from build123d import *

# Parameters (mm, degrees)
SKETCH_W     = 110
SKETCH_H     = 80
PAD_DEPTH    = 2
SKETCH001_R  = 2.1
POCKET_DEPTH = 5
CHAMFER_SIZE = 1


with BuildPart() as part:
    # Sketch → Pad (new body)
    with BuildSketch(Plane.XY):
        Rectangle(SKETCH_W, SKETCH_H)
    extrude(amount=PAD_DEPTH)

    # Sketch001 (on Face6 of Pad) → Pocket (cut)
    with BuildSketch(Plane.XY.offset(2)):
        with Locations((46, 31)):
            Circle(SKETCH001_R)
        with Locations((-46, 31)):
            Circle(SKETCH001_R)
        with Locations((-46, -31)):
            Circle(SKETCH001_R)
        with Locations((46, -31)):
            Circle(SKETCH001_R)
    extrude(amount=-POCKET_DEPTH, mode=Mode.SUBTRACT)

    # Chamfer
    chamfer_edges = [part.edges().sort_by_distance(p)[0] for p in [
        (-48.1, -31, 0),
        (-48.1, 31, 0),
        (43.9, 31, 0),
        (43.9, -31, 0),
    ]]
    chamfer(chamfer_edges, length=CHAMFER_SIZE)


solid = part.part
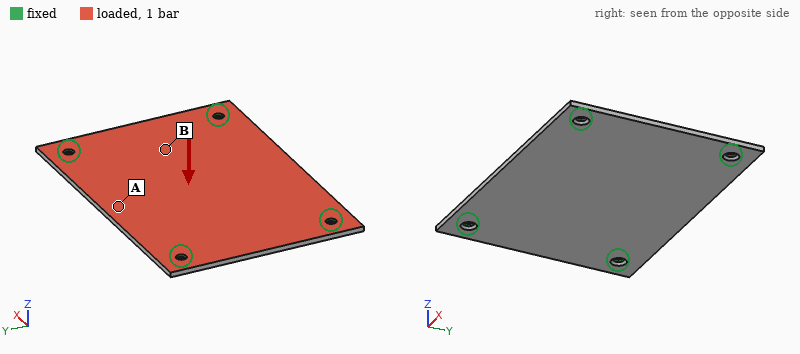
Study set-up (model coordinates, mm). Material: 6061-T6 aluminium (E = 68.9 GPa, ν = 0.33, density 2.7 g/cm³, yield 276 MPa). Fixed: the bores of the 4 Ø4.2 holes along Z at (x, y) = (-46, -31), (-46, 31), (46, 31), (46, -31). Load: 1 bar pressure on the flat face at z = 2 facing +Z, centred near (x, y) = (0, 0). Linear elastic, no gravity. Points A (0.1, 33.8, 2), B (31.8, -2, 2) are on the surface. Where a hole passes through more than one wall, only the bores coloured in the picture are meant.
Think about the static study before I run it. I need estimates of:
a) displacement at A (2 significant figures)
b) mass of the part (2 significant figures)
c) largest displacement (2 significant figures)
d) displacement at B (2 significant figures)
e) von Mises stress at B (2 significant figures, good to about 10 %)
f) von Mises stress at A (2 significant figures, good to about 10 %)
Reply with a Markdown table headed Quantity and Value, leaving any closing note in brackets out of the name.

| Quantity | Value |
|---|---|
| displacement at A | 0.57 mm |
| mass of the part | 47 g |
| largest displacement | 0.65 mm |
| displacement at B | 0.34 mm |
| von Mises stress at B | 31 MPa |
| von Mises stress at A | 64 MPa |
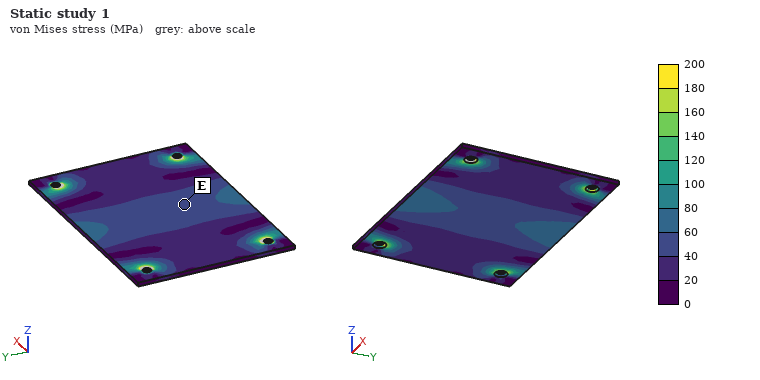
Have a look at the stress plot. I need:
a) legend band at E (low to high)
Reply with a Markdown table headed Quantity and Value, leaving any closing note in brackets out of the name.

| Quantity | Value |
|---|---|
| legend band at E | 40 to 60 MPa |
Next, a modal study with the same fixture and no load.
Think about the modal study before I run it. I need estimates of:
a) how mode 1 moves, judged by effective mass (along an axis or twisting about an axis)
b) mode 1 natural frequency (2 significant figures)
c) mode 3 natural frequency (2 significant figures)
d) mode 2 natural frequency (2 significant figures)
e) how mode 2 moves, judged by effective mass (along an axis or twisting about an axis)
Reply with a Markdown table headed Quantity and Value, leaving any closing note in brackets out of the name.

| Quantity | Value |
|---|---|
| how mode 1 moves, judged by effective mass | along Z |
| mode 1 natural frequency | 990 Hz |
| mode 3 natural frequency | 2300 Hz |
| mode 2 natural frequency | 1500 Hz |
| how mode 2 moves, judged by effective mass | twisting about X |
